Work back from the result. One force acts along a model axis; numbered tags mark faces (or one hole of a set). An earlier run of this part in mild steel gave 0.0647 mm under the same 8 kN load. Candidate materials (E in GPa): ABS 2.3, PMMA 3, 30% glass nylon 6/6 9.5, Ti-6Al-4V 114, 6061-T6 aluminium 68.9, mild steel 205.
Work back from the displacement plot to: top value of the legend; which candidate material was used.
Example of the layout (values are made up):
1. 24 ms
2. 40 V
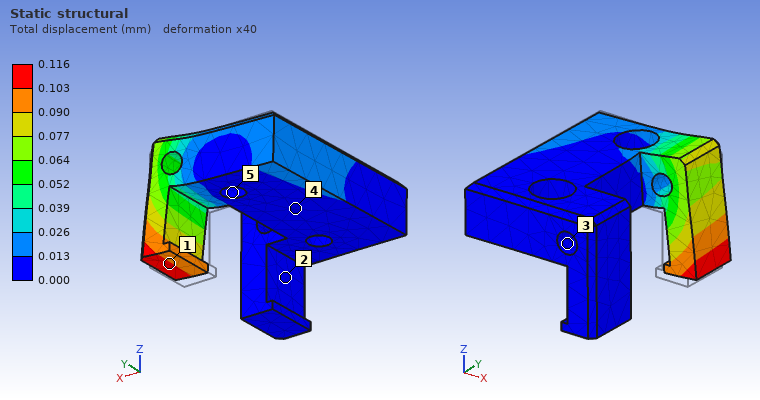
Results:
1. 0.116 mm
2. Ti-6Al-4V
